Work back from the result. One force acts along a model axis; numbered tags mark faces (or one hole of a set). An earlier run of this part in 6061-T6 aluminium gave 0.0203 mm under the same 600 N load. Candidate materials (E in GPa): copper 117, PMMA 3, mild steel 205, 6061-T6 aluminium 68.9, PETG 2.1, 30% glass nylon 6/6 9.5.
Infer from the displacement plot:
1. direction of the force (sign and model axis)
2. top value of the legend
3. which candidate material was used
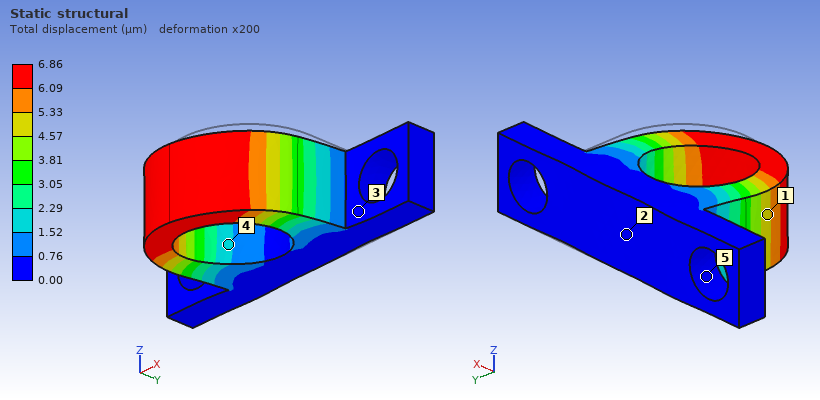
-X
6.86 µm
mild steel
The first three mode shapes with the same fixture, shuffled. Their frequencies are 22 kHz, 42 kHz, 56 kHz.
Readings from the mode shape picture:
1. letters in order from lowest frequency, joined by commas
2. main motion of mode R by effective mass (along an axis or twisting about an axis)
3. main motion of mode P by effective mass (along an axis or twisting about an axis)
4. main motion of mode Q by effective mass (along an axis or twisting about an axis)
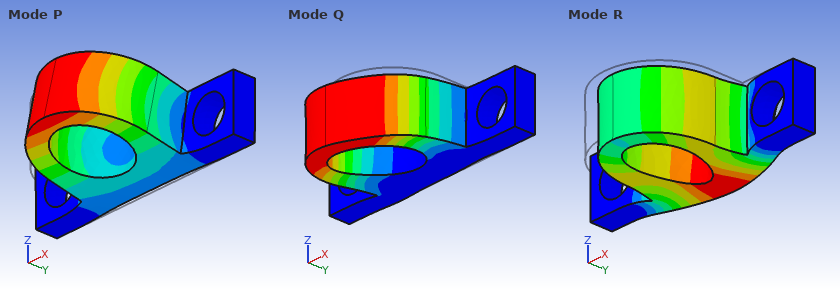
P, Q, R
along Y
along Z
along X
